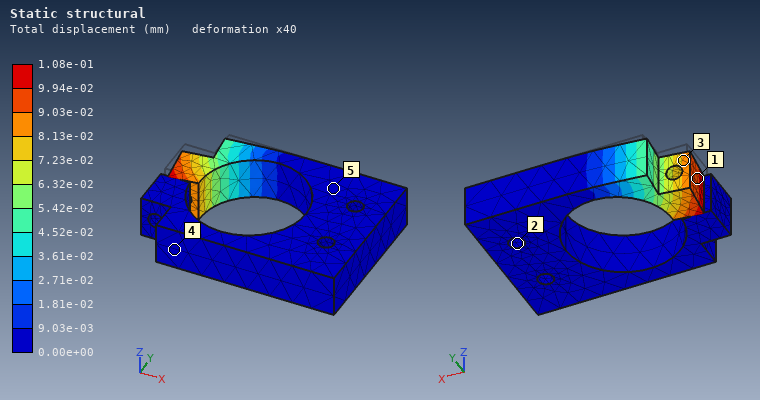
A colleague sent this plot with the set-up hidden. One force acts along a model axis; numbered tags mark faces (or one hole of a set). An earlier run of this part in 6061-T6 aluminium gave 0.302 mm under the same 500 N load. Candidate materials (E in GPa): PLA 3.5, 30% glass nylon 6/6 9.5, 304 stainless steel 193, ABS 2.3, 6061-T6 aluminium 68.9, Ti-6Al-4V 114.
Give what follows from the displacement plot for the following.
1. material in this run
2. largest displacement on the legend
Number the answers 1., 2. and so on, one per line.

1. 304 stainless steel
2. 1.08e-01 mm
